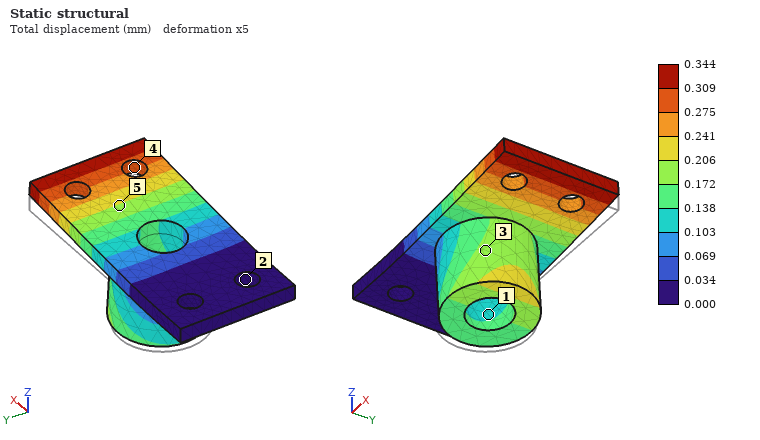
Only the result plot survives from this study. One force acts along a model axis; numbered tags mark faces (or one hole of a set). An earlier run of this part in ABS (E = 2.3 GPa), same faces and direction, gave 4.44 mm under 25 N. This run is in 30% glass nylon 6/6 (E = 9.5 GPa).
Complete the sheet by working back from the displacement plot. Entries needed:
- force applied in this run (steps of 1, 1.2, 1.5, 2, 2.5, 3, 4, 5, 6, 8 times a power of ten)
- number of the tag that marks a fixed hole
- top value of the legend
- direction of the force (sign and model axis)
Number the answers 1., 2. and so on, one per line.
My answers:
1. 8 N
2. 2
3. 0.344 mm
4. +Z
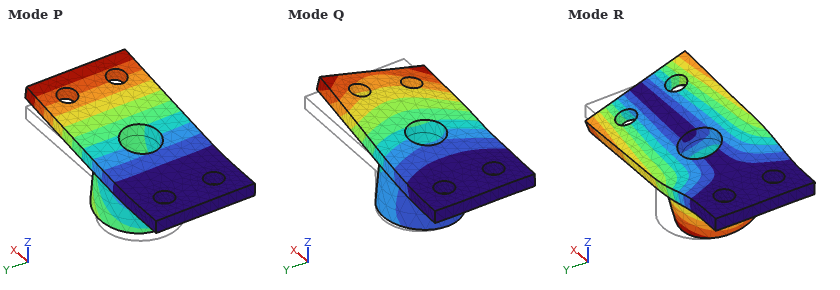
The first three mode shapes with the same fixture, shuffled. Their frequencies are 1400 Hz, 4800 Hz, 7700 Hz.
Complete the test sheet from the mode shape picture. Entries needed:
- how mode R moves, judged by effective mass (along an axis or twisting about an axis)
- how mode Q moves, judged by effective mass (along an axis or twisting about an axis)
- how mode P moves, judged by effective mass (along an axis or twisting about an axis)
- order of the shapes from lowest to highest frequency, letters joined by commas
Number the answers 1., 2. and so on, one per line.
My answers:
1. along Y
2. along Y
3. along Z
4. P, R, Q
